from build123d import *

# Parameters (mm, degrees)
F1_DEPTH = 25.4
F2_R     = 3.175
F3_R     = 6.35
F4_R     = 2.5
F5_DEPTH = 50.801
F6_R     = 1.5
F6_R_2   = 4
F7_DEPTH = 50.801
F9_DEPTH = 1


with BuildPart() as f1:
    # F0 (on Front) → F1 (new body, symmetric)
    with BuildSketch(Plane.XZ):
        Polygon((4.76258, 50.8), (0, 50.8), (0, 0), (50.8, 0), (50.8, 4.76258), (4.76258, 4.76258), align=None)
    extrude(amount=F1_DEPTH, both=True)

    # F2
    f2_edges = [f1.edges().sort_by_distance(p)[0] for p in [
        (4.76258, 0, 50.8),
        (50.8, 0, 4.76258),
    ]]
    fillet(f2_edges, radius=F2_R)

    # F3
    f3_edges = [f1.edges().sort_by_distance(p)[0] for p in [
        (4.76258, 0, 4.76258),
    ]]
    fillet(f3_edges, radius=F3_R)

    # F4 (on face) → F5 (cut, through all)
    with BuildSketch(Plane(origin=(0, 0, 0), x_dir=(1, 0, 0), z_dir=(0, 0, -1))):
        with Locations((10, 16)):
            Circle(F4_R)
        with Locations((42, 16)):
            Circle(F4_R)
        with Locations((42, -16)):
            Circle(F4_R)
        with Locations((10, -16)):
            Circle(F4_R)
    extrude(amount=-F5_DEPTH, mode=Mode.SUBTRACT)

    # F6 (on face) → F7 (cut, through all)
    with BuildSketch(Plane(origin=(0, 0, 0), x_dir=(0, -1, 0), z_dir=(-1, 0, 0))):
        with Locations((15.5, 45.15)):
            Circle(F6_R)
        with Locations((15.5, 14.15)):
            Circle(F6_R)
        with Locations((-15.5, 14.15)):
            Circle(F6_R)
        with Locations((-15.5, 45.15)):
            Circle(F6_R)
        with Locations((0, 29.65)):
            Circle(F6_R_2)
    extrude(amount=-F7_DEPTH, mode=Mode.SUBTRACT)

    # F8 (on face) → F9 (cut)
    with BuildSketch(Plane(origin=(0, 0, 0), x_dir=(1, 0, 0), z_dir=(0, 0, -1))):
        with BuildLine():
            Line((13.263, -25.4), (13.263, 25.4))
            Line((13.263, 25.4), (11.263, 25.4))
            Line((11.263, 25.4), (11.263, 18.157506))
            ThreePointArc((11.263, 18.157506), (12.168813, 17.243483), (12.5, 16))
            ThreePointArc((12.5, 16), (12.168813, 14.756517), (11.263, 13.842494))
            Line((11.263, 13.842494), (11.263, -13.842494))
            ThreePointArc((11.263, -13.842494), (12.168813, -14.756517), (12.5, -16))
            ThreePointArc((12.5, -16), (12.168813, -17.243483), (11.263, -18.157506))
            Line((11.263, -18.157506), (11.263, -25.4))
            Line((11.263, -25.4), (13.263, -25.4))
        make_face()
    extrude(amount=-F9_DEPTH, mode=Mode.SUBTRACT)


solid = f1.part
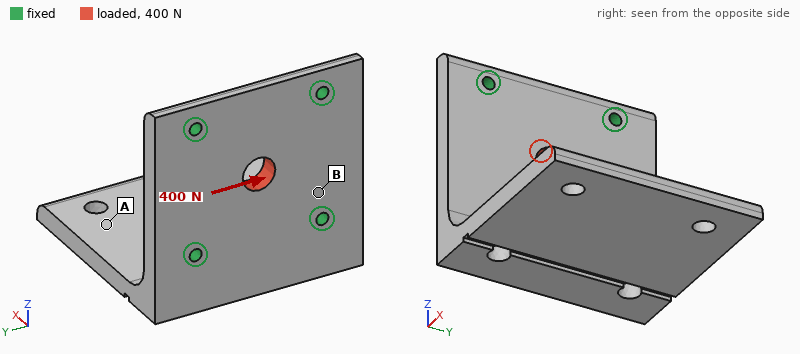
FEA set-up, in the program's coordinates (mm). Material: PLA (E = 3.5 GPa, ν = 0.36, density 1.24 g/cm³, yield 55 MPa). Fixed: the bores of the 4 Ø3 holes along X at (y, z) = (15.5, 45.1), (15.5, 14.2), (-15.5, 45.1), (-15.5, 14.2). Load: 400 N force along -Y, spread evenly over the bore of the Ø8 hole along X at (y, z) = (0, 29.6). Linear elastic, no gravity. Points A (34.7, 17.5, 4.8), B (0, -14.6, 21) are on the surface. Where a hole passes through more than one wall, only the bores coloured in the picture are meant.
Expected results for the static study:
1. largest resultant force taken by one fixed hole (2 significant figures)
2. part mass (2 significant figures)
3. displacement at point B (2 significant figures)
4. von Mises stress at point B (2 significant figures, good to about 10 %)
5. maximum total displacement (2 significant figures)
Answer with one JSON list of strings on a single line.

["110 N", "28 g", "6.2 µm", "1.5 MPa", "16 µm"]
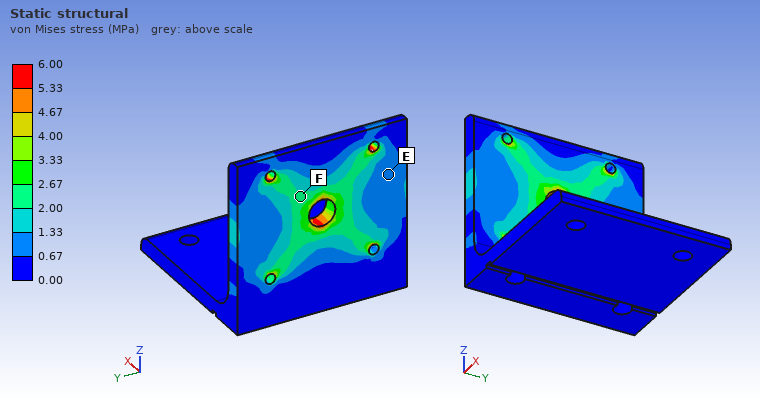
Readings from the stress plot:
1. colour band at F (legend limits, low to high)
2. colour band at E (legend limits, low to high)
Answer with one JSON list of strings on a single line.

["2.00 to 2.67 MPa", "0.67 to 1.33 MPa"]
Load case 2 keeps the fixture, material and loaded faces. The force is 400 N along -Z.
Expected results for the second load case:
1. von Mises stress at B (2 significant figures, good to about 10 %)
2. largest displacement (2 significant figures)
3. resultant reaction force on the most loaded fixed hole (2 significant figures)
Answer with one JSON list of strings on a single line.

["1.4 MPa", "17 µm", "110 N"]
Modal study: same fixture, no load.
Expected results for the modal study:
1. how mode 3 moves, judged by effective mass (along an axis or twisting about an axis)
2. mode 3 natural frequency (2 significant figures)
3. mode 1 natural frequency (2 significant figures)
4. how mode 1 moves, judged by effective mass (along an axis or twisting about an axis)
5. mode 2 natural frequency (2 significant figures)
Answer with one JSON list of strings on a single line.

["along Y", "1600 Hz", "440 Hz", "along Z", "1100 Hz"]
